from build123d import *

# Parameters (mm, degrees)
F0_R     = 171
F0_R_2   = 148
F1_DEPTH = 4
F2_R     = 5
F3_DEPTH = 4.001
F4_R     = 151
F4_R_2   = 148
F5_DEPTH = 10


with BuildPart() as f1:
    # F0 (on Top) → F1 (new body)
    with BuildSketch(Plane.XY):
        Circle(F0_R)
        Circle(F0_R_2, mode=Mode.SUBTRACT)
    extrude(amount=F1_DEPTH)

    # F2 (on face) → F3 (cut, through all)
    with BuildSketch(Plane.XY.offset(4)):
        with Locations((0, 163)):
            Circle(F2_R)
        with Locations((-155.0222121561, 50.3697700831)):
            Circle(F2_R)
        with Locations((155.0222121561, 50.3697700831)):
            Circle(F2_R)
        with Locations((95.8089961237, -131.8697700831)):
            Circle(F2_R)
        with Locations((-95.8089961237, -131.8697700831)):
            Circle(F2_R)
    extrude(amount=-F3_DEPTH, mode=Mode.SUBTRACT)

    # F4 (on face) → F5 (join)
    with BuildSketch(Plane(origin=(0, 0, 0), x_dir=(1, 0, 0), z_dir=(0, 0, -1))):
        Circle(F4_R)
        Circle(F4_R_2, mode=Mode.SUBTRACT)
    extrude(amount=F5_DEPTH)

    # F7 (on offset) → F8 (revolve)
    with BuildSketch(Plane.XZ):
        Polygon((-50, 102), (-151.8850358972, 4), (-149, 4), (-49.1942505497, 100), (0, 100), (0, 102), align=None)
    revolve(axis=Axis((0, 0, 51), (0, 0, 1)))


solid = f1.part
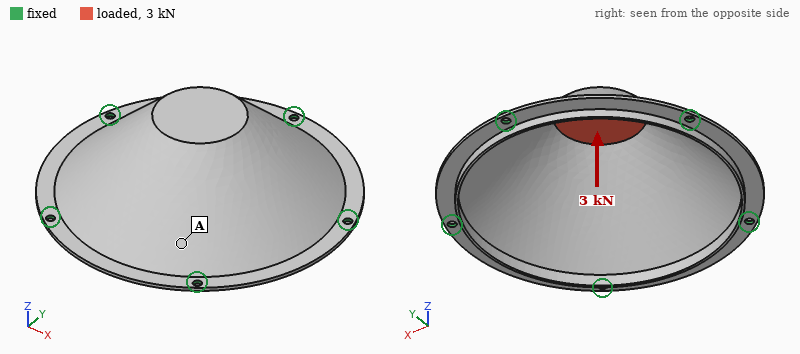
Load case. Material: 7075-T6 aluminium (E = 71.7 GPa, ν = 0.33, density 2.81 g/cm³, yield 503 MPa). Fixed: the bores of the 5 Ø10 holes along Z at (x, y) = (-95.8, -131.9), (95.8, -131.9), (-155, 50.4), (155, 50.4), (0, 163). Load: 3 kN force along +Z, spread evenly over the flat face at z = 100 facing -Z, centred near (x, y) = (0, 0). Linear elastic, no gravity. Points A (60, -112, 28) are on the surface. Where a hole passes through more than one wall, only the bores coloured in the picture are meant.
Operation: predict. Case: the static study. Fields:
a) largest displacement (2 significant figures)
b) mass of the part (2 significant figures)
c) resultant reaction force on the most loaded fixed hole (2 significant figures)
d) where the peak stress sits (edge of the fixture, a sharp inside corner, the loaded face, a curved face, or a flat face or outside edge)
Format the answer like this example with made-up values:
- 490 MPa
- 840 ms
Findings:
- 0.94 mm
- 870 g
- 860 N
- a flat face or outside edge
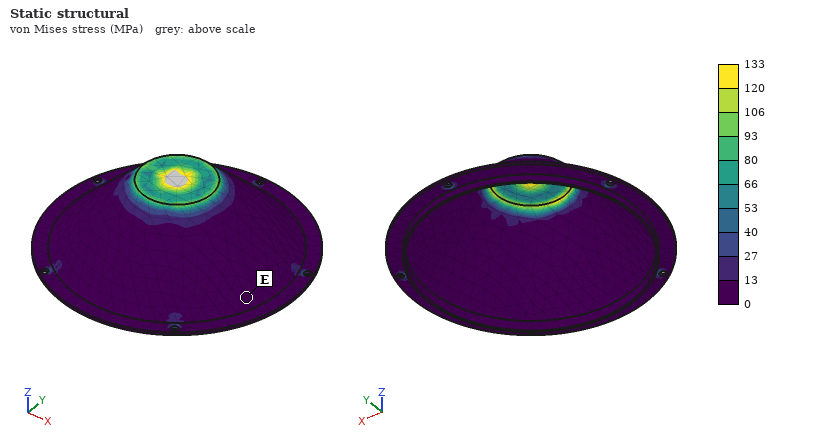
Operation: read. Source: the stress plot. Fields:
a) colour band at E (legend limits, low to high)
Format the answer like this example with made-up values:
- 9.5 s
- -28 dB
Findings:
- 0 to 13 MPa
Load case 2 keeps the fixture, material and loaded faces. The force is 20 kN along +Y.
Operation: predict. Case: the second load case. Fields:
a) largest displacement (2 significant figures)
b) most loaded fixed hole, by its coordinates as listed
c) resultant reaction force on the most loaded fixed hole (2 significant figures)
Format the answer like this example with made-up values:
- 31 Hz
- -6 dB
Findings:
- 0.32 mm
- (0, 163)
- 7.5 kN
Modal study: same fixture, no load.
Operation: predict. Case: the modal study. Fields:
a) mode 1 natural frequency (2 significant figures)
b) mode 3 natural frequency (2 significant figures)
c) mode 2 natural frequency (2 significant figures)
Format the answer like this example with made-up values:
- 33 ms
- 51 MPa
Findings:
- 1700 Hz
- 1700 Hz
- 1700 Hz
